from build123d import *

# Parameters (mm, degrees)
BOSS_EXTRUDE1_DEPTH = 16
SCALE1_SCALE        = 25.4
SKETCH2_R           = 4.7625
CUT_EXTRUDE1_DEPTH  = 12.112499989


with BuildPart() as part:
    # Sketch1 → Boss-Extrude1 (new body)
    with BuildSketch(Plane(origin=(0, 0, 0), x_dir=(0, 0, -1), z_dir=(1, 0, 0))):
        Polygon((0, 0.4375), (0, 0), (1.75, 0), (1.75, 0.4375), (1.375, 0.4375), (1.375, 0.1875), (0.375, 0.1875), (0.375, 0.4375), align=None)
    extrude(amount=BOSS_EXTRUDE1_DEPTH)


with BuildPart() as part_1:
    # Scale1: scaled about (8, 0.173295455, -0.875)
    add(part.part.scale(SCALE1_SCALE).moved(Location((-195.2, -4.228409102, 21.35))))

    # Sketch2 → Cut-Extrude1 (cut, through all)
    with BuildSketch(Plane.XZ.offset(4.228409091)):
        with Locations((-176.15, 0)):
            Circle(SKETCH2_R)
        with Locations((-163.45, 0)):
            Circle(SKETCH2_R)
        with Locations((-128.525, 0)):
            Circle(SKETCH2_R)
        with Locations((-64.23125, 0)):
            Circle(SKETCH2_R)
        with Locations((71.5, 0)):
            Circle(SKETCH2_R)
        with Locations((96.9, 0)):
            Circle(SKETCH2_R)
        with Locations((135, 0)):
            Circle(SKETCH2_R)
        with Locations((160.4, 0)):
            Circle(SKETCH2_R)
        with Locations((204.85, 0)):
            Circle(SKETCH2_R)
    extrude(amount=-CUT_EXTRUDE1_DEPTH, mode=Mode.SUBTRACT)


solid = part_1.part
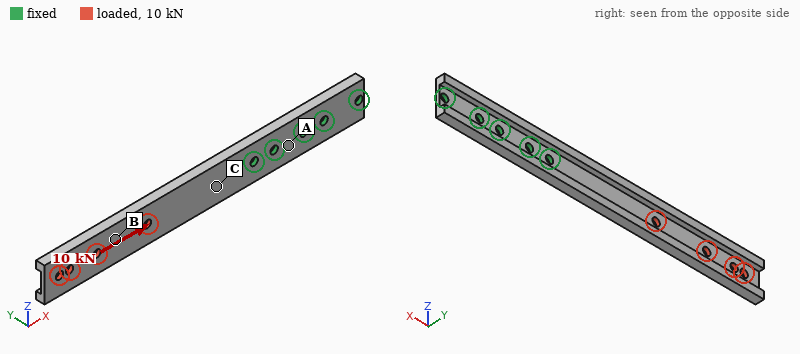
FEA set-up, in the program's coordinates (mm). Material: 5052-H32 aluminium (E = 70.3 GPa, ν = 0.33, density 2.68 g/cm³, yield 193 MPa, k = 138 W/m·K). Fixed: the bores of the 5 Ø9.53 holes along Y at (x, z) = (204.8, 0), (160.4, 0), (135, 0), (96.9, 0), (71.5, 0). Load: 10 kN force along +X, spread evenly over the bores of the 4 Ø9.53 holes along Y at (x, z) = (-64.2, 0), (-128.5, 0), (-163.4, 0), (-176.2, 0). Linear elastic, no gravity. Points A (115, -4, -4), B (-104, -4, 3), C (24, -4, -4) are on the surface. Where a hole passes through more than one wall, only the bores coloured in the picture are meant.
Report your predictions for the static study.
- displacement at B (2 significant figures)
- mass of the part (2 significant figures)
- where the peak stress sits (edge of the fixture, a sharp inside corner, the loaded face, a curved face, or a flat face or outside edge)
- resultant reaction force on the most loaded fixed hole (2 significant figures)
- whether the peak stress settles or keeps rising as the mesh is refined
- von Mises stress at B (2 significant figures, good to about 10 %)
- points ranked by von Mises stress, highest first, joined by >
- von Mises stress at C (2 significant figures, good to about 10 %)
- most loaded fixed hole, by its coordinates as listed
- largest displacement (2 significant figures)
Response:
1.4 mm
350 g
edge of the fixture
7.2 kN
keeps rising
43 MPa
C > B > A
58 MPa
(71.5, 0)
2.9 mm
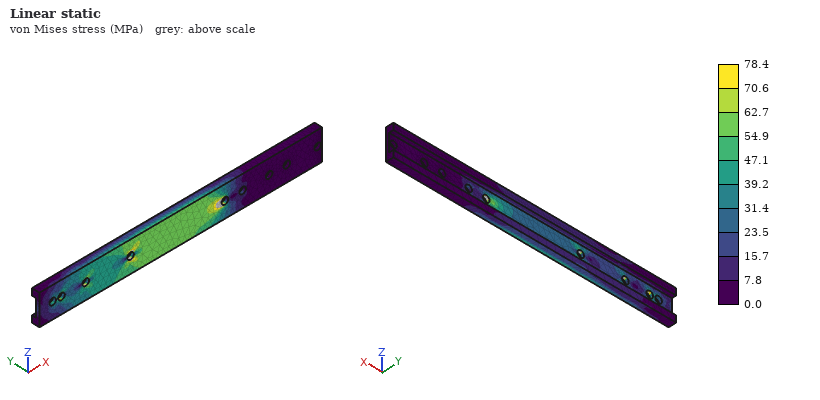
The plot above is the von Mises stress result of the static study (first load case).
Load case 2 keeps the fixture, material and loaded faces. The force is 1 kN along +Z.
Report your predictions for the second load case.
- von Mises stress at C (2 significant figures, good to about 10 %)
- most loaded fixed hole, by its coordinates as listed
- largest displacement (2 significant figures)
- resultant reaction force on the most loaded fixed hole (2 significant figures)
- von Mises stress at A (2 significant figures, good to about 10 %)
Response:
9.9 MPa
(71.5, 0)
1.2 mm
4.5 kN
13 MPa
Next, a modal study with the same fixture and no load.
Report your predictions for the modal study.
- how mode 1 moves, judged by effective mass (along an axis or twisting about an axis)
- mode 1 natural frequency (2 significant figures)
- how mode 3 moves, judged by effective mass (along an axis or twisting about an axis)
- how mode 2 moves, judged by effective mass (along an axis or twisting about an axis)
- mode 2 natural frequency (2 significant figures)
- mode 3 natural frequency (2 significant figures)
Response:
along Y
120 Hz
twisting about X
along Z
480 Hz
720 Hz
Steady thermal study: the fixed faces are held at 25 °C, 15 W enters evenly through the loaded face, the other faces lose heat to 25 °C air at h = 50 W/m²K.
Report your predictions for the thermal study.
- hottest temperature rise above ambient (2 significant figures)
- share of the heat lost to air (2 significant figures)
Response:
18 K
88 %
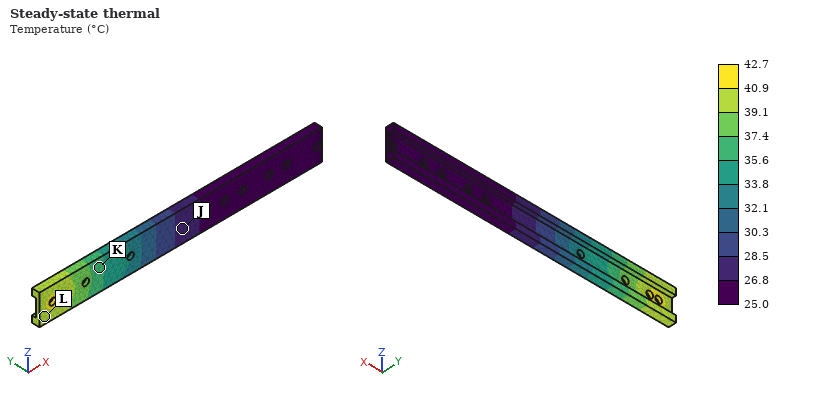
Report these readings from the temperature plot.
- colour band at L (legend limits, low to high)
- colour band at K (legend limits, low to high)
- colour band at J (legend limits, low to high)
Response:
39.1 to 40.9 °C
35.6 to 37.4 °C
26.8 to 28.5 °C
